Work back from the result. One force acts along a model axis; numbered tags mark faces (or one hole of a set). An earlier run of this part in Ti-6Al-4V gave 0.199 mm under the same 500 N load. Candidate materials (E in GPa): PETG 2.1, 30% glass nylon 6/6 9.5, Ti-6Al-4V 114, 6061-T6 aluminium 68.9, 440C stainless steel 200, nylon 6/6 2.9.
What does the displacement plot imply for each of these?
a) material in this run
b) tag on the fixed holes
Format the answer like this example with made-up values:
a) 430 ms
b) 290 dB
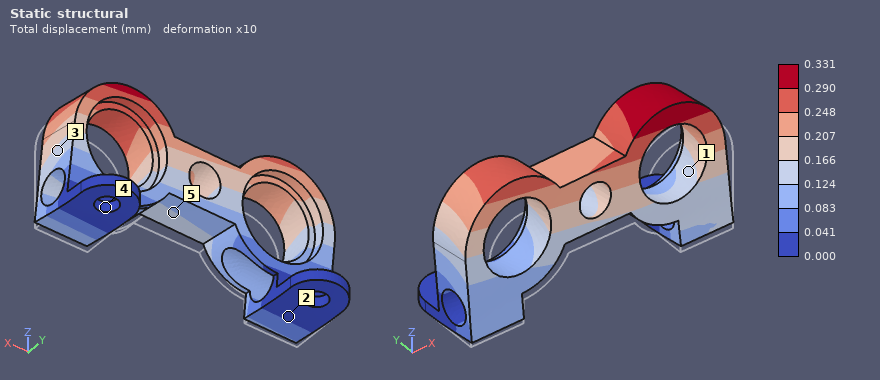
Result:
a) 6061-T6 aluminium
b) 4
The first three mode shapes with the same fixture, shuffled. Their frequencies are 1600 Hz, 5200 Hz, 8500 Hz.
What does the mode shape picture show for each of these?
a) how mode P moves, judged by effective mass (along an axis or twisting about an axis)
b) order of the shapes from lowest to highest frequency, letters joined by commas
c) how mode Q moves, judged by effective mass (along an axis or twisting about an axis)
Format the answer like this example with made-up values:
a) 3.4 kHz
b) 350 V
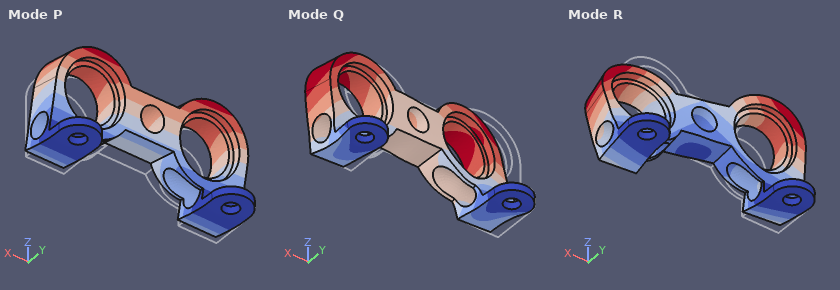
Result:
a) along Y
b) P, R, Q
c) along X
